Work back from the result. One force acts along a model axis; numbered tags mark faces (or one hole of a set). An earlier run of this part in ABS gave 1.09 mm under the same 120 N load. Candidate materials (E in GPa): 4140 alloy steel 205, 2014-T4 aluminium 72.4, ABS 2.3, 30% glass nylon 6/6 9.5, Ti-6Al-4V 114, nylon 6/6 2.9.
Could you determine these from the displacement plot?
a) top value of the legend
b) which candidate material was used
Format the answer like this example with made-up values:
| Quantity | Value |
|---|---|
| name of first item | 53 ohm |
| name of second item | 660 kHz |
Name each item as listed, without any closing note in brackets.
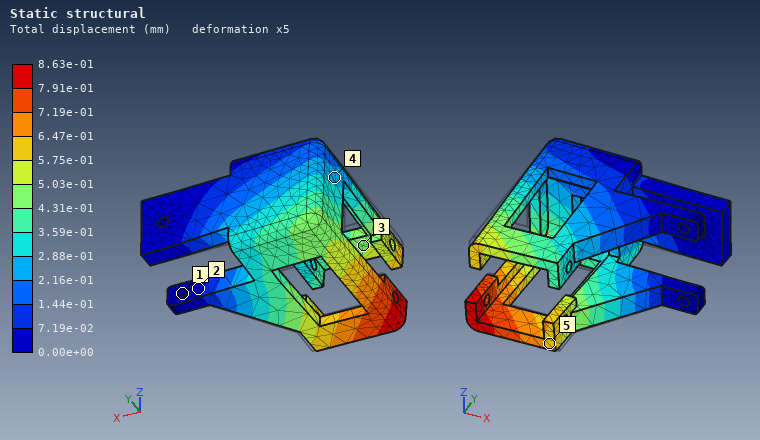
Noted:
| Quantity | Value |
|---|---|
| top value of the legend | 8.63e-01 mm |
| which candidate material was used | nylon 6/6 |
